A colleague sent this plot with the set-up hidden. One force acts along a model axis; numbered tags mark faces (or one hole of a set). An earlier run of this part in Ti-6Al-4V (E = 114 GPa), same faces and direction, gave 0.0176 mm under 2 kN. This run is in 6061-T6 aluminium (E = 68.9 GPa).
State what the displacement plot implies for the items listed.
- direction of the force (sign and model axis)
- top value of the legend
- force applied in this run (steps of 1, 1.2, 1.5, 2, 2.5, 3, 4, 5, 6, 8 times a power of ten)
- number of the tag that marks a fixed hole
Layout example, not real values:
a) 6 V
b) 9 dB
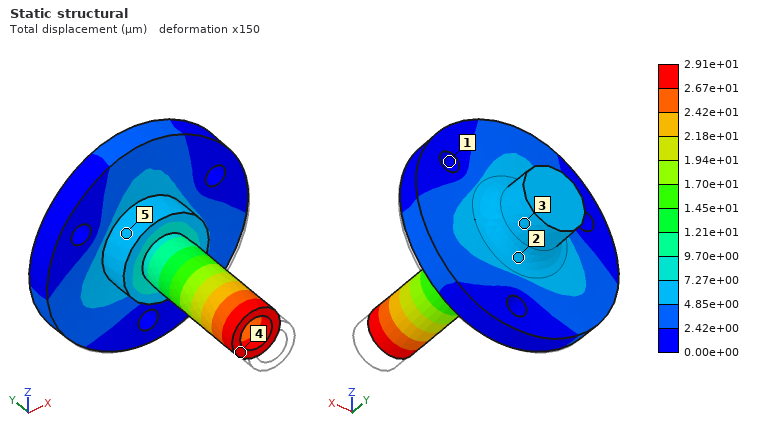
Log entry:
a) +Y
b) 2.91e+01 µm
c) 2 kN
d) 1
